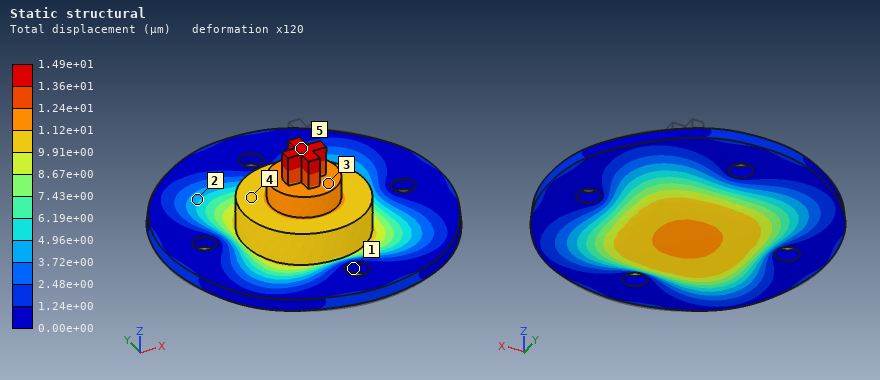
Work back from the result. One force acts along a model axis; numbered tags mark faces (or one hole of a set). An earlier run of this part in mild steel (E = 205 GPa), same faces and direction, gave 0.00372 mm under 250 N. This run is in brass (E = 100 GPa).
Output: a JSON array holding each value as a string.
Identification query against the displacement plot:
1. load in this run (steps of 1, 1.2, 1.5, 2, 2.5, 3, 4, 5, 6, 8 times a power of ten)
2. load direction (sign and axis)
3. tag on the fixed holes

["500 N", "-Z", "1"]
